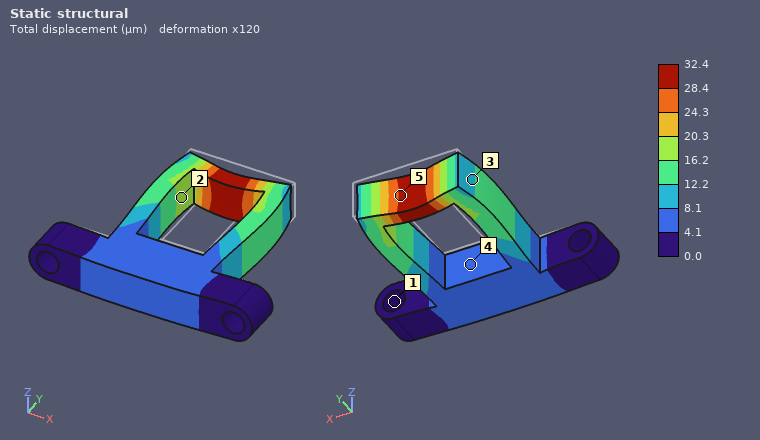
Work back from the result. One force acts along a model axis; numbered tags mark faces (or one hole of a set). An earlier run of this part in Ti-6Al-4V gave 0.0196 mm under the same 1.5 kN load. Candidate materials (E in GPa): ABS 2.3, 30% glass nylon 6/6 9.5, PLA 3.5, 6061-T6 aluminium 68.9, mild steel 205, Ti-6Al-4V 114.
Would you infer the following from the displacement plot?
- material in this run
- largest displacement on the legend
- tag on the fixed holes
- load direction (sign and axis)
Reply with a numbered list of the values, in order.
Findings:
1. 6061-T6 aluminium
2. 32.4 µm
3. 1
4. -Y
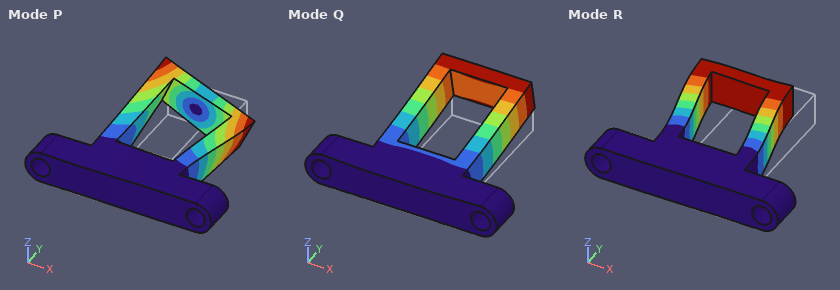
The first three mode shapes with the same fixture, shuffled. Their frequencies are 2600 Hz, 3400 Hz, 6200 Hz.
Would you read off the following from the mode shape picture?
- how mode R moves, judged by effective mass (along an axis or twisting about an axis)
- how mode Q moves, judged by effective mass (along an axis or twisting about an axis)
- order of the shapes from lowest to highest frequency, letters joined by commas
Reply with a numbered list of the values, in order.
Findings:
1. along X
2. along Z
3. Q, R, P
